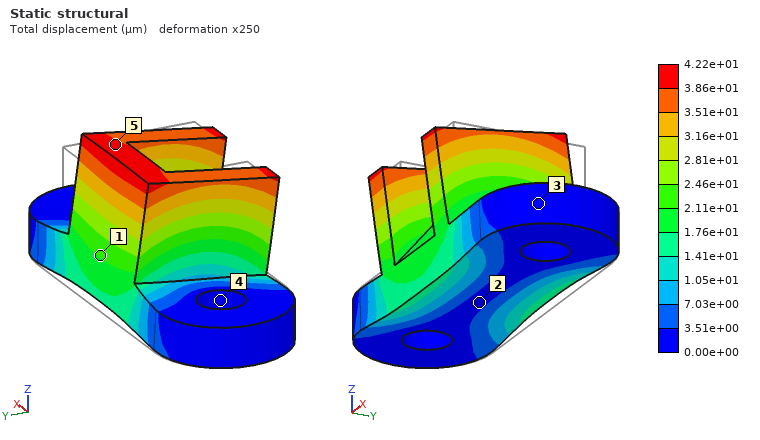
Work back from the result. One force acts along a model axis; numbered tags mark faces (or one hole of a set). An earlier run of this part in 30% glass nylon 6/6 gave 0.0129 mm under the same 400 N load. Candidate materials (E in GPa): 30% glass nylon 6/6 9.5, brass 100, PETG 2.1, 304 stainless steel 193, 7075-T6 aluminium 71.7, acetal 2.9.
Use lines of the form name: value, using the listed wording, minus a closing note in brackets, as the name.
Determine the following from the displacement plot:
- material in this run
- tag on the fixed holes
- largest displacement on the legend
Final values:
material in this run: acetal
tag on the fixed holes: 4
largest displacement on the legend: 4.22e+01 µm
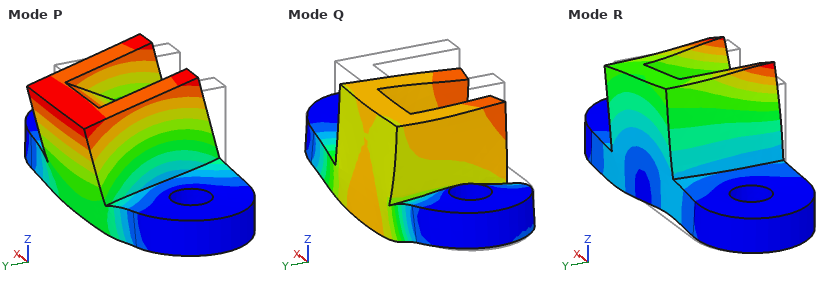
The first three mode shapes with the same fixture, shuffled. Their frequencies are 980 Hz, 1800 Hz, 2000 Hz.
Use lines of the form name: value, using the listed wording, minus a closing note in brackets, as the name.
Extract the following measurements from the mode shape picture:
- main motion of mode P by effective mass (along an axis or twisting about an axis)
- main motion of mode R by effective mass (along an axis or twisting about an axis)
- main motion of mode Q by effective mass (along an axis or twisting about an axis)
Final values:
main motion of mode P by effective mass: along Y
main motion of mode R by effective mass: along X
main motion of mode Q by effective mass: along Z
